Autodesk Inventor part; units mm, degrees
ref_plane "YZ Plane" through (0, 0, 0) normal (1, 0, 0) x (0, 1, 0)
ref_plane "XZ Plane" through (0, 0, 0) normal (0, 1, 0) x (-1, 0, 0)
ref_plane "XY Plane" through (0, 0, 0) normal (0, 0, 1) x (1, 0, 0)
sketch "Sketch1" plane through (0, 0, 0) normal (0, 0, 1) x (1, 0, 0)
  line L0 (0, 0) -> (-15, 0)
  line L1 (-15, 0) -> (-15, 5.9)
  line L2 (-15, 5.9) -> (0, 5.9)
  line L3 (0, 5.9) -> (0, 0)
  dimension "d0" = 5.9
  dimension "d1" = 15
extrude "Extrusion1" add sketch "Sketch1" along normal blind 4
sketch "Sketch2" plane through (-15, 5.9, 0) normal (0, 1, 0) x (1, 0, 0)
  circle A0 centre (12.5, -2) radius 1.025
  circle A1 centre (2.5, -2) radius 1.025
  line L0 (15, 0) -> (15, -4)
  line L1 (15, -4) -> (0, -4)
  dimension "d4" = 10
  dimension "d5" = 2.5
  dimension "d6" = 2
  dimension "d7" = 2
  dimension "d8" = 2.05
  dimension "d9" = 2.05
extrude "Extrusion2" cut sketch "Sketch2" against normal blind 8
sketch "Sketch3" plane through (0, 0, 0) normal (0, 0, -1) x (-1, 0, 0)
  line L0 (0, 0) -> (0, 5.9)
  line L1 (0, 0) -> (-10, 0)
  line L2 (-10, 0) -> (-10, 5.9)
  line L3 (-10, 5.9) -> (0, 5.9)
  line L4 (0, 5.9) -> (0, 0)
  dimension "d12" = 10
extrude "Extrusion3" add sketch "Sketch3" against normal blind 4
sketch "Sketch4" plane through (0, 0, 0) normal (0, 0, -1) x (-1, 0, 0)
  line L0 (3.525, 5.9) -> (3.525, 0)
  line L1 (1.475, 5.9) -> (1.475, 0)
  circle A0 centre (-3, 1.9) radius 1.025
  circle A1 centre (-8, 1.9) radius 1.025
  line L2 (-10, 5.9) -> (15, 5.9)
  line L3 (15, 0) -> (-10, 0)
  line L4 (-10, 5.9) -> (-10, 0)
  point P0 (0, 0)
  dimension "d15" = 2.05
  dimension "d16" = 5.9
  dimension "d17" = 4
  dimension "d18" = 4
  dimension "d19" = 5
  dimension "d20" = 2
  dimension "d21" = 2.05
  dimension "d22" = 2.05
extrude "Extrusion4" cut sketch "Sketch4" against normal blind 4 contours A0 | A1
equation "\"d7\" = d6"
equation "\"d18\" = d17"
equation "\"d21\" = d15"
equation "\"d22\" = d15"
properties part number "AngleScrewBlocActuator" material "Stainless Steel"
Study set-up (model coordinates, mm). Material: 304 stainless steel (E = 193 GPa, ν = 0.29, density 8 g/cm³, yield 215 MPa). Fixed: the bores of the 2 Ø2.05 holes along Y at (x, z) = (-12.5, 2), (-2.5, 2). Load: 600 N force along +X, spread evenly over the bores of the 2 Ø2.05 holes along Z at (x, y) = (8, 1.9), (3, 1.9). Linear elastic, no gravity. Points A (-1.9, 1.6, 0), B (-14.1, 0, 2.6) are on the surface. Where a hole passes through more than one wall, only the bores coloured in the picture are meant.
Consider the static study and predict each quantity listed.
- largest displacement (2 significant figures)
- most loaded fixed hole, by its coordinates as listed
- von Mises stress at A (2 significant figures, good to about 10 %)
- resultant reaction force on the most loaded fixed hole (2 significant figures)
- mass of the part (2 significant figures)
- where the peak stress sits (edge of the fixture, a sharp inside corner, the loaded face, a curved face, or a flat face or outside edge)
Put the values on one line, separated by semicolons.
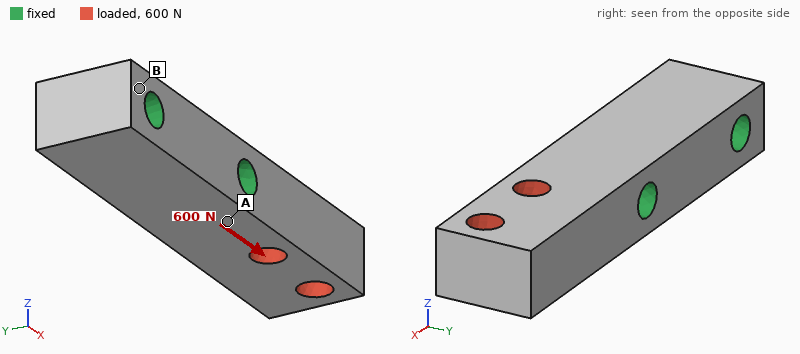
4.4 µm; (-2.5, 2); 20 MPa; 590 N; 4.2 g; the loaded face
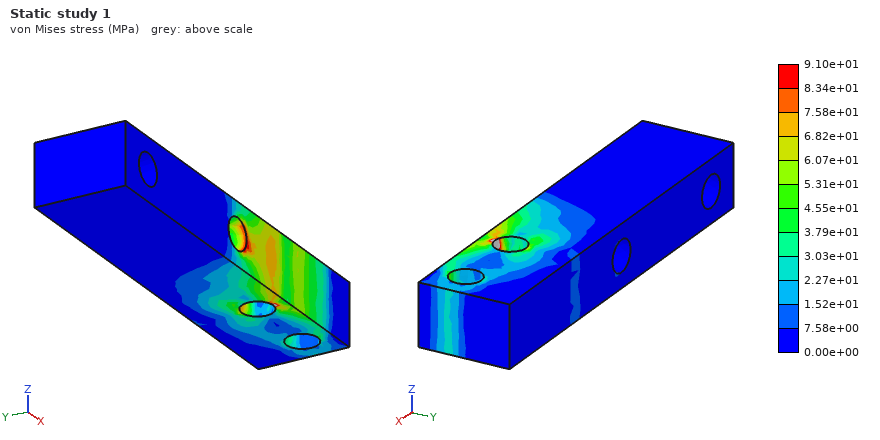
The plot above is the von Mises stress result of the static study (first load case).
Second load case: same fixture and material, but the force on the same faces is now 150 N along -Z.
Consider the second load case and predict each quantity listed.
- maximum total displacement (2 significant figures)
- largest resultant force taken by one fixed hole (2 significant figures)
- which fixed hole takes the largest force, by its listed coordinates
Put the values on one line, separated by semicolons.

11 µm; 170 N; (-2.5, 2)
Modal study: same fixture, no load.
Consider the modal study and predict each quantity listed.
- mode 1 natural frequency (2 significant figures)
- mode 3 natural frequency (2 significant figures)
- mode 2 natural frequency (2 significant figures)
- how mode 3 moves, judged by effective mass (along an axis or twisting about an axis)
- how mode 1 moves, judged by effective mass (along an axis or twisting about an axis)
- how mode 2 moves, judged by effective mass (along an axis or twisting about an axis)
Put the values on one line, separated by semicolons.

19 kHz; 53 kHz; 28 kHz; twisting about X; along Z; along Y
